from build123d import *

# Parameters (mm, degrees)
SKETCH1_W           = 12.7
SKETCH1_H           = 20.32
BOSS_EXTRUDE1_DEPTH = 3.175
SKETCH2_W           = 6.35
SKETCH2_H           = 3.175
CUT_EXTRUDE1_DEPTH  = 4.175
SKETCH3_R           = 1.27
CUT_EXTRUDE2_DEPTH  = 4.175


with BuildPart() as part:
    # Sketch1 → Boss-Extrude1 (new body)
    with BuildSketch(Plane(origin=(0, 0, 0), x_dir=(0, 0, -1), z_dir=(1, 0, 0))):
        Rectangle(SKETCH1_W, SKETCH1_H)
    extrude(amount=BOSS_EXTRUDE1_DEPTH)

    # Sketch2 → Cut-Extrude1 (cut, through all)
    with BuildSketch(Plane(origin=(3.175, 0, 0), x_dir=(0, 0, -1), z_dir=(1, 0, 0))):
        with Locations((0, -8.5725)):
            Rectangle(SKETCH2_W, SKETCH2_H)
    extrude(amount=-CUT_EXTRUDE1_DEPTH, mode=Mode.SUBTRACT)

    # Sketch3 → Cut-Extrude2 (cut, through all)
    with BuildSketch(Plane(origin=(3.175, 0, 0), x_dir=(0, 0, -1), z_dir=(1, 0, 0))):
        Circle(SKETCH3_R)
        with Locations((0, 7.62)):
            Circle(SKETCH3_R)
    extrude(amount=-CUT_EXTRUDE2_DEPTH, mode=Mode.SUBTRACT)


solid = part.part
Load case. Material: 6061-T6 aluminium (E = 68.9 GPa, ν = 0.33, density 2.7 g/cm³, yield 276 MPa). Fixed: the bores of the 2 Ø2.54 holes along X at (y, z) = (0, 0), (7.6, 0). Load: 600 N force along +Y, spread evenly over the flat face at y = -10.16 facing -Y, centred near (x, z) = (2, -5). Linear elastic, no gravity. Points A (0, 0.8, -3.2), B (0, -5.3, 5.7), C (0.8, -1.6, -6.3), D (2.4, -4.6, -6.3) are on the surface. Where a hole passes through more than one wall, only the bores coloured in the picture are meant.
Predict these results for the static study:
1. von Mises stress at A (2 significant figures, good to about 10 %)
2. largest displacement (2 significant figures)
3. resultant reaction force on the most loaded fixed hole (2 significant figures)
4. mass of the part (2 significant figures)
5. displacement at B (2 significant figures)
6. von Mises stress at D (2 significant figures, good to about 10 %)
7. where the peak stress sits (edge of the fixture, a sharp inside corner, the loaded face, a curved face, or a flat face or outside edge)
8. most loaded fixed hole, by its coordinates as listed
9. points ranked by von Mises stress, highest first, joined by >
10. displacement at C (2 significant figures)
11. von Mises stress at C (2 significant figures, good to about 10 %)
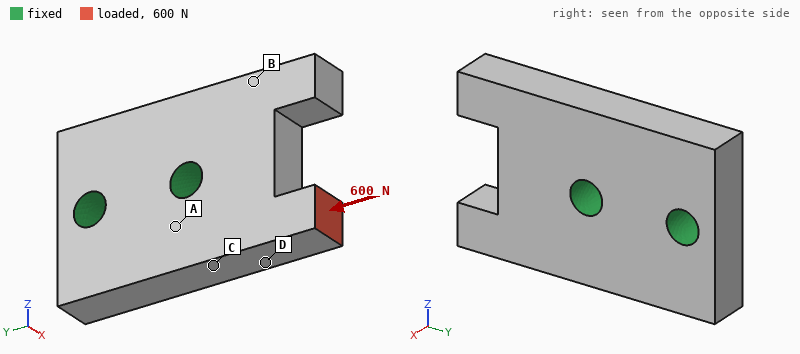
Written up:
32 MPa
18 µm
510 N
2.0 g
3.6 µm
68 MPa
edge of the fixture
(0, 0)
D > C > A > B
5.6 µm
52 MPa
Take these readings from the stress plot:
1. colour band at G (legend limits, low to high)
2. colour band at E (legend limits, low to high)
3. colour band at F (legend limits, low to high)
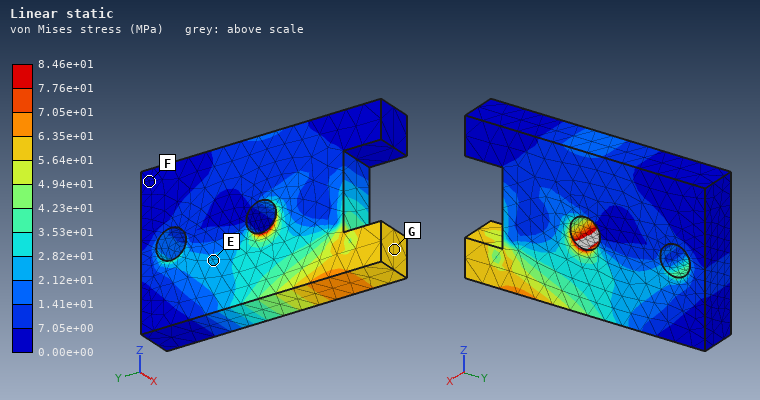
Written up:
5.64e+01 to 6.35e+01 MPa
2.12e+01 to 2.82e+01 MPa
0.00e+00 to 7.05e+00 MPa
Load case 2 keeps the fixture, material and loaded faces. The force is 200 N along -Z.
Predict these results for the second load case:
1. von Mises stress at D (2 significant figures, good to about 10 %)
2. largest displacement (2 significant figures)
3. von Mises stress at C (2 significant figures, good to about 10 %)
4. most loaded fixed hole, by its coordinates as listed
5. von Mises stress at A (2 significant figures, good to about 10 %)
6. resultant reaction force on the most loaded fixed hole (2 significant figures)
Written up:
73 MPa
26 µm
39 MPa
(0, 0)
16 MPa
370 N
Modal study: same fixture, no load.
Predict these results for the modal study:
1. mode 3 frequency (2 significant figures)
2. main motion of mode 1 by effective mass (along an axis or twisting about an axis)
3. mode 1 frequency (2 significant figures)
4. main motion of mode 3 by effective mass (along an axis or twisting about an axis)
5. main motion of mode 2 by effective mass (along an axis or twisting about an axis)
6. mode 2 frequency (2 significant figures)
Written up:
45 kHz
along X
28 kHz
along Z
twisting about Y
31 kHz
